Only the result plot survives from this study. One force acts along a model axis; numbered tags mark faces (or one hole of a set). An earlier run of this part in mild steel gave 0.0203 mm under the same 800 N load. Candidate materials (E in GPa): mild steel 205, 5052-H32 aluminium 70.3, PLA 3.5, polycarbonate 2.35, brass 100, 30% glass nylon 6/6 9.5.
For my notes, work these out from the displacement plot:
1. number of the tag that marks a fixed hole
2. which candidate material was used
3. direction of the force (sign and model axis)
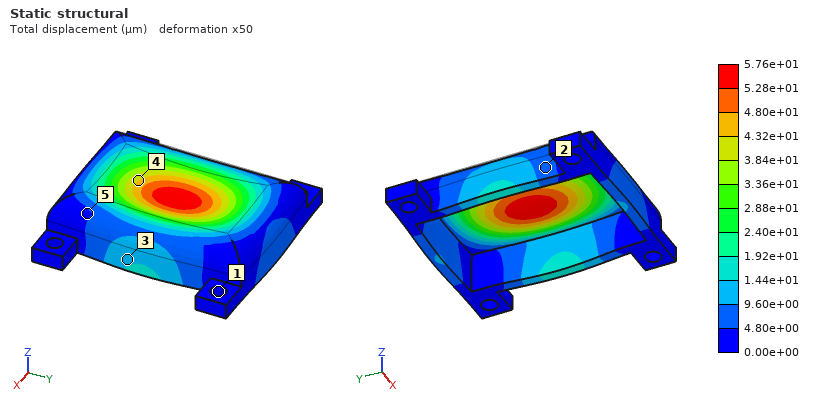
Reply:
1
5052-H32 aluminium
-Z
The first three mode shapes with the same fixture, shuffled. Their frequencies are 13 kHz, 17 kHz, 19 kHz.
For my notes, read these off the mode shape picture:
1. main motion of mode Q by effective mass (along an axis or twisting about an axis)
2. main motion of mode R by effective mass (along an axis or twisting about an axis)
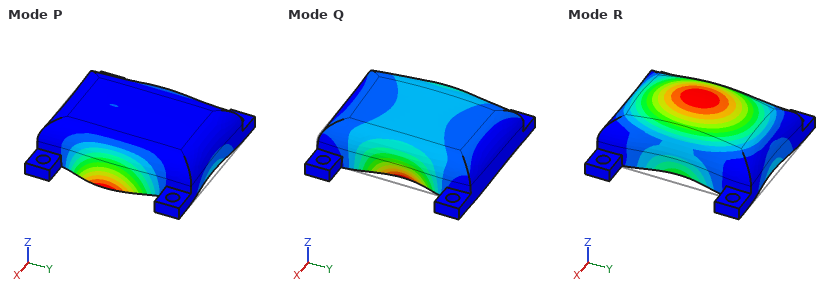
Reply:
along X
along Z
